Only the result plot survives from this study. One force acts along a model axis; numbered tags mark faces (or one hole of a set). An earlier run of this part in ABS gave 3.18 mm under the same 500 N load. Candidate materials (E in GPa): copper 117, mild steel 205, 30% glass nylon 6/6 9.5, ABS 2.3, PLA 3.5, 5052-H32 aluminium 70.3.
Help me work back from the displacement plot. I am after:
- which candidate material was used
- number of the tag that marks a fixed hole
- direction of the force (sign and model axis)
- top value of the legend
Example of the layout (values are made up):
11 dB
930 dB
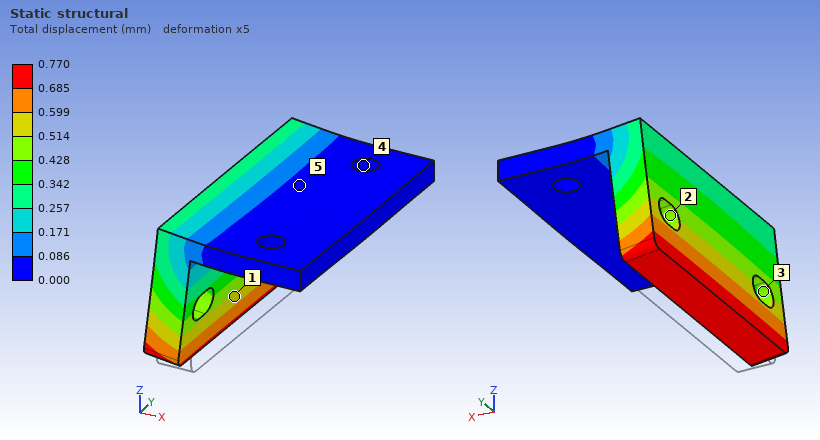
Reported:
30% glass nylon 6/6
4
-X
0.770 mm
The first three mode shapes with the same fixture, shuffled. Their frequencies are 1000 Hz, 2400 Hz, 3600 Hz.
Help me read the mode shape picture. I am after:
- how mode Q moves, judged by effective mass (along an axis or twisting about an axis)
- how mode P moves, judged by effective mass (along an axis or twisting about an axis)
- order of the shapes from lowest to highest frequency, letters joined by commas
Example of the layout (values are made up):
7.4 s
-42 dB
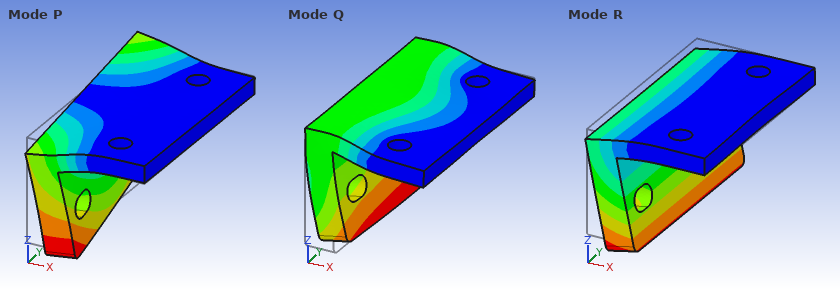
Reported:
along Z
along Y
R, P, Q
